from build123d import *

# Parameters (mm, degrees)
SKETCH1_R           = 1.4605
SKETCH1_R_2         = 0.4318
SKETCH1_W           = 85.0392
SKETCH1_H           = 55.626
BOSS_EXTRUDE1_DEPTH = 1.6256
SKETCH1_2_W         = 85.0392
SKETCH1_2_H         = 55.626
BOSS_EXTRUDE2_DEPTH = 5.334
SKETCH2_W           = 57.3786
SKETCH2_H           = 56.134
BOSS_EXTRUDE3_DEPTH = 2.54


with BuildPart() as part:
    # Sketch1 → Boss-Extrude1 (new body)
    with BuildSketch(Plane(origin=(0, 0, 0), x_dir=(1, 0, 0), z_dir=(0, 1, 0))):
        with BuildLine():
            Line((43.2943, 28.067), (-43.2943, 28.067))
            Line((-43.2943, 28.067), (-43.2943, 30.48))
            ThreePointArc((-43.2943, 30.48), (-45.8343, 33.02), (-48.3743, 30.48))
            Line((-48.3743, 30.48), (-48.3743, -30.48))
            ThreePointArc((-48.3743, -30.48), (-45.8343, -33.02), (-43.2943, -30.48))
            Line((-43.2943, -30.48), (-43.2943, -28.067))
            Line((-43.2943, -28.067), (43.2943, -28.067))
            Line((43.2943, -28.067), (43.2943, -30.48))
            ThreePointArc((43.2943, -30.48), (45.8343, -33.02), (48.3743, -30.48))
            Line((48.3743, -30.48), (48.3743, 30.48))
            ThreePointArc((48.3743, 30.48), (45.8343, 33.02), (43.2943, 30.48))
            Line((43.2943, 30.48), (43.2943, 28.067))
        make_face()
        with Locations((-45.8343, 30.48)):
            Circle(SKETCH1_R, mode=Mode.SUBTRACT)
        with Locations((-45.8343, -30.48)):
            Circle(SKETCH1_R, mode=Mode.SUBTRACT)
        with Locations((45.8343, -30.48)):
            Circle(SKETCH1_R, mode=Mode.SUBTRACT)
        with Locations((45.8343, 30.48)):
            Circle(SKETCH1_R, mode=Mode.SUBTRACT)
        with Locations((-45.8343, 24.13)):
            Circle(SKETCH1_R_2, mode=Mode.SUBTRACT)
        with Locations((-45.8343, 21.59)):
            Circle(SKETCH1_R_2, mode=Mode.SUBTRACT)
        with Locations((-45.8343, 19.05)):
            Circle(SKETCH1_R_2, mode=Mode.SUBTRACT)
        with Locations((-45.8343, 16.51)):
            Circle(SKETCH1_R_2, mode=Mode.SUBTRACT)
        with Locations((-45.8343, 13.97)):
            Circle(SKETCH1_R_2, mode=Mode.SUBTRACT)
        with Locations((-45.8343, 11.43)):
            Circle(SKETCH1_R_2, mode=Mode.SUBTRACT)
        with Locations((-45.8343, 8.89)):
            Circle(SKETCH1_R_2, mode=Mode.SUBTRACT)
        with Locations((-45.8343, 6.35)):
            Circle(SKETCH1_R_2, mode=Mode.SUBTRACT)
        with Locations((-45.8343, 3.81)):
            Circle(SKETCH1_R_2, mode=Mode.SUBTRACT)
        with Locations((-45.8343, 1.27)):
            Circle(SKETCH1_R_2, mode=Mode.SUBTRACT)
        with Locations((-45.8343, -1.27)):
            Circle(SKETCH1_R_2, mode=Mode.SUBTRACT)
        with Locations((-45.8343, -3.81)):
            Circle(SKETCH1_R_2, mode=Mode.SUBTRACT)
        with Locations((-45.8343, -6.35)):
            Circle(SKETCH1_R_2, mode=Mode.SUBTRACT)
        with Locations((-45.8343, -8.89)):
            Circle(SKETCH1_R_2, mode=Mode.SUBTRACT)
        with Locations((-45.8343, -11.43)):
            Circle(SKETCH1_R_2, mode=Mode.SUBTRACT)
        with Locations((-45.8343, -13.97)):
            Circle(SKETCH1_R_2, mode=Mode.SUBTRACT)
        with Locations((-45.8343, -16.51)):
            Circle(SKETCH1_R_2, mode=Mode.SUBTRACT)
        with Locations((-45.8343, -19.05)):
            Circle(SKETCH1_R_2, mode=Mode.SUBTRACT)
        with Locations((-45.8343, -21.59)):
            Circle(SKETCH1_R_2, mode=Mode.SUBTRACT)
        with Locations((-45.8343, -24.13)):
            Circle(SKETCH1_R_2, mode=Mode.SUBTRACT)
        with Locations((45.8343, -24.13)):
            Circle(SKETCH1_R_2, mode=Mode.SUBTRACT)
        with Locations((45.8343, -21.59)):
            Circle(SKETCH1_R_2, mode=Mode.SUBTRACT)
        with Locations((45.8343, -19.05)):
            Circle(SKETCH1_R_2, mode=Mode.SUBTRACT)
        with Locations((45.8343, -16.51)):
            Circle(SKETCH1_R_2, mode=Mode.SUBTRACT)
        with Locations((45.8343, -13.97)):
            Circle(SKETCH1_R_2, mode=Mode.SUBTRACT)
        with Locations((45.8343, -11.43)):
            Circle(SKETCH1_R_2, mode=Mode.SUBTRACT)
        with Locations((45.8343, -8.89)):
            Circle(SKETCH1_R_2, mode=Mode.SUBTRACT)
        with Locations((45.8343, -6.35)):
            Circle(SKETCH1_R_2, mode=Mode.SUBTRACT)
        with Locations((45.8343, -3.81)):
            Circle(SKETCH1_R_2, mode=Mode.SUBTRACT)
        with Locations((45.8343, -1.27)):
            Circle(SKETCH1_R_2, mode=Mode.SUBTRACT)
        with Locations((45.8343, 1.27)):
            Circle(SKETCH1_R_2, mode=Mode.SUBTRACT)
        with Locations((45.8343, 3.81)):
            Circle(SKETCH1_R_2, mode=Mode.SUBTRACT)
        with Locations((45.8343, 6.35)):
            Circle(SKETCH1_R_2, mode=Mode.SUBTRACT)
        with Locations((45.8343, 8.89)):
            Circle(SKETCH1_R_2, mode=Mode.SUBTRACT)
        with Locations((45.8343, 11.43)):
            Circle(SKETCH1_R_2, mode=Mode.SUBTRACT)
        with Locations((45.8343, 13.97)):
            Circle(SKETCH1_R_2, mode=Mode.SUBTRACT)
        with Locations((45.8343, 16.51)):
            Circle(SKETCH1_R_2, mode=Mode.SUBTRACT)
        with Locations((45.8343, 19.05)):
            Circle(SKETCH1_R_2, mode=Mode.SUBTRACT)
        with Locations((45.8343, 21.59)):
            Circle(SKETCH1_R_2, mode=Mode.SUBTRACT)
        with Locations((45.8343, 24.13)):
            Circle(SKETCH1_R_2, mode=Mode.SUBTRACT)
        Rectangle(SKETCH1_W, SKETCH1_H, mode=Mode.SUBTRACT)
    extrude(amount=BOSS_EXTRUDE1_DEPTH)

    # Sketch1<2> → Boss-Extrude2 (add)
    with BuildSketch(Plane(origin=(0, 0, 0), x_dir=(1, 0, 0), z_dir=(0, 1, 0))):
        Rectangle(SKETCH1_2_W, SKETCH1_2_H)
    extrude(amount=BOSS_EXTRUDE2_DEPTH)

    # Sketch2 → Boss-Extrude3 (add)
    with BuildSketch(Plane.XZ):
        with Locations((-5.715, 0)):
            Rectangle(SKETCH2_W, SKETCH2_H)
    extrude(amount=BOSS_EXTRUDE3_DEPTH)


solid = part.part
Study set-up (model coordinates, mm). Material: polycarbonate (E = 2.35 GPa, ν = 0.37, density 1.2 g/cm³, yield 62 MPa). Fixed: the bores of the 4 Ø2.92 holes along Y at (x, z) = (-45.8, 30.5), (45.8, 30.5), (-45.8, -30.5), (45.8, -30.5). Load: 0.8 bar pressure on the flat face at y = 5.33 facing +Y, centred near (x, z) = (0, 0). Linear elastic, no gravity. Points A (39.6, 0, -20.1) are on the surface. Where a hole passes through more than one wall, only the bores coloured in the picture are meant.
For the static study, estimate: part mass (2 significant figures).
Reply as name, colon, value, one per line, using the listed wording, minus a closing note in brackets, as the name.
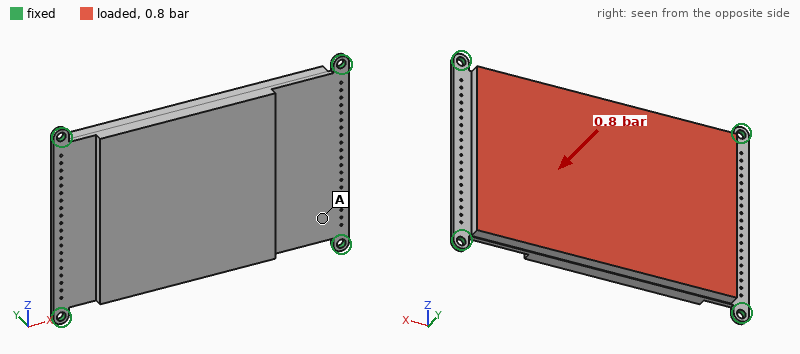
part mass: 42 g
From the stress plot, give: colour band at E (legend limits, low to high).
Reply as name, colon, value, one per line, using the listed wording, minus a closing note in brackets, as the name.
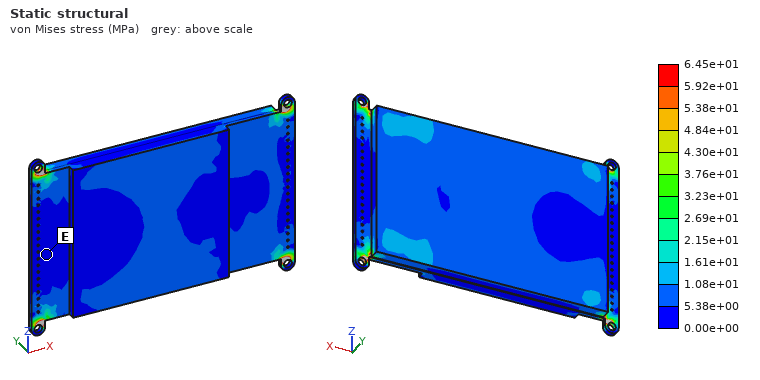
colour band at E: 0.00e+00 to 5.38e+00 MPa
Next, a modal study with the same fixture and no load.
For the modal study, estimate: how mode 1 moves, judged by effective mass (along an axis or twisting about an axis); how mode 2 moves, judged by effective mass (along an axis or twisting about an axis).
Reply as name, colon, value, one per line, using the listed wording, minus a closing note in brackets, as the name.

how mode 1 moves, judged by effective mass: along Y
how mode 2 moves, judged by effective mass: twisting about X
